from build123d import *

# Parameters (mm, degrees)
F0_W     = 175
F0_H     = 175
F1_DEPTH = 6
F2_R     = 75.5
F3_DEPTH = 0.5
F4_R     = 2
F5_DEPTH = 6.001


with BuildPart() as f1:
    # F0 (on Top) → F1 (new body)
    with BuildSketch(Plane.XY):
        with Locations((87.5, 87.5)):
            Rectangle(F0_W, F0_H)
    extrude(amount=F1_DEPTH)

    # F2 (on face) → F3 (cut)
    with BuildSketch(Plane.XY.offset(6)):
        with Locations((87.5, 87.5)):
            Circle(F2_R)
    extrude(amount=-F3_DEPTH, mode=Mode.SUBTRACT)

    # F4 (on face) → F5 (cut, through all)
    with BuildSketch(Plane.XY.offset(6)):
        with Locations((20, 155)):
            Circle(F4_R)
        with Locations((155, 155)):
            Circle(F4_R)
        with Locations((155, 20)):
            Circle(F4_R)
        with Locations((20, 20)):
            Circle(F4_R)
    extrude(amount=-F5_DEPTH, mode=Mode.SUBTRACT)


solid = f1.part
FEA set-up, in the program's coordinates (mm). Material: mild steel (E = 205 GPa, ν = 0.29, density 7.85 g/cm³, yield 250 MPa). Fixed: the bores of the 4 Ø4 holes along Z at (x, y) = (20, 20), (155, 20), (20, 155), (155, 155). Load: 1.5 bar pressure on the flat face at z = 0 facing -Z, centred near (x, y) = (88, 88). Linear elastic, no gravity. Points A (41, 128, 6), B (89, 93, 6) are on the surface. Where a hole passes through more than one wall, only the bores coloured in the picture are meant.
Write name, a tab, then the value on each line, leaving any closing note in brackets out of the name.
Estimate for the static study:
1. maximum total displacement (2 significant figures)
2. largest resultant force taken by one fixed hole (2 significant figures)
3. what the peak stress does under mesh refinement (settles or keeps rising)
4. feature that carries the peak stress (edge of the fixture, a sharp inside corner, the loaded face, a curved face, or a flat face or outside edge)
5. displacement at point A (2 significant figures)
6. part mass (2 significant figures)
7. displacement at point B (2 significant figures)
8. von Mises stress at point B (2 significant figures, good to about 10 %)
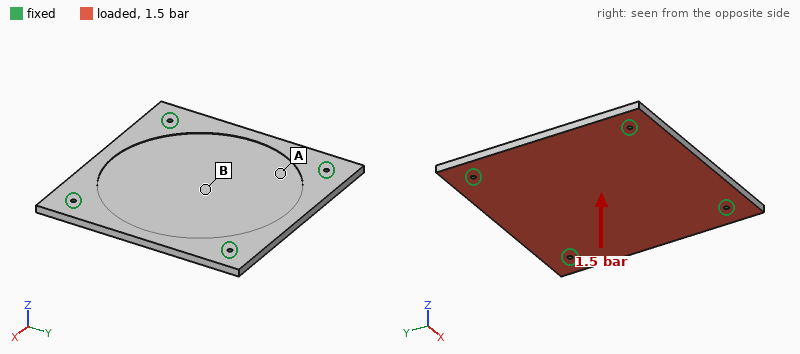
maximum total displacement	0.12 mm
largest resultant force taken by one fixed hole	1.2 kN
what the peak stress does under mesh refinement	keeps rising
feature that carries the peak stress	edge of the fixture
displacement at point A	0.057 mm
part mass	1.4 kg
displacement at point B	0.12 mm
von Mises stress at point B	28 MPa
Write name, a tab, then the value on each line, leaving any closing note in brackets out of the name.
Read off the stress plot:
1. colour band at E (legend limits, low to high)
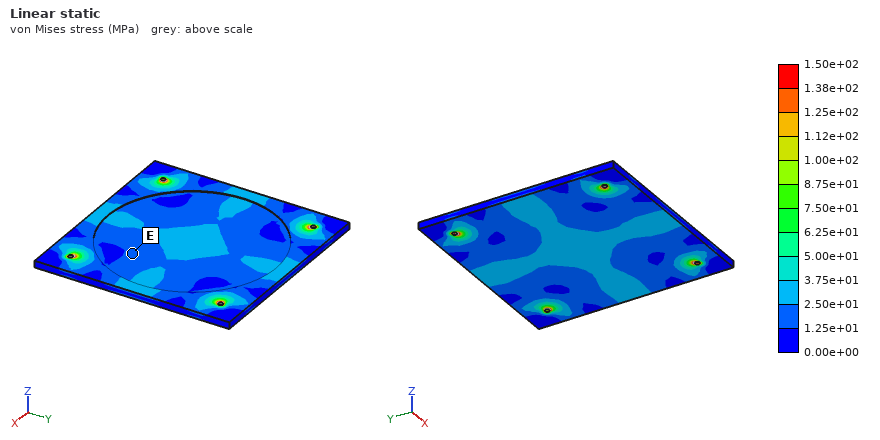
colour band at E	1.25e+01 to 2.50e+01 MPa
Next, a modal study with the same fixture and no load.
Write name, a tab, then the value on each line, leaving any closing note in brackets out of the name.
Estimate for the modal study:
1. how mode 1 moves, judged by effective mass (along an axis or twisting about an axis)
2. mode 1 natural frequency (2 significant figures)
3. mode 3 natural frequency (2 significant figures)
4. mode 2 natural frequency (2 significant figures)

how mode 1 moves, judged by effective mass	along Z
mode 1 natural frequency	1000 Hz
mode 3 natural frequency	1700 Hz
mode 2 natural frequency	1700 Hz
